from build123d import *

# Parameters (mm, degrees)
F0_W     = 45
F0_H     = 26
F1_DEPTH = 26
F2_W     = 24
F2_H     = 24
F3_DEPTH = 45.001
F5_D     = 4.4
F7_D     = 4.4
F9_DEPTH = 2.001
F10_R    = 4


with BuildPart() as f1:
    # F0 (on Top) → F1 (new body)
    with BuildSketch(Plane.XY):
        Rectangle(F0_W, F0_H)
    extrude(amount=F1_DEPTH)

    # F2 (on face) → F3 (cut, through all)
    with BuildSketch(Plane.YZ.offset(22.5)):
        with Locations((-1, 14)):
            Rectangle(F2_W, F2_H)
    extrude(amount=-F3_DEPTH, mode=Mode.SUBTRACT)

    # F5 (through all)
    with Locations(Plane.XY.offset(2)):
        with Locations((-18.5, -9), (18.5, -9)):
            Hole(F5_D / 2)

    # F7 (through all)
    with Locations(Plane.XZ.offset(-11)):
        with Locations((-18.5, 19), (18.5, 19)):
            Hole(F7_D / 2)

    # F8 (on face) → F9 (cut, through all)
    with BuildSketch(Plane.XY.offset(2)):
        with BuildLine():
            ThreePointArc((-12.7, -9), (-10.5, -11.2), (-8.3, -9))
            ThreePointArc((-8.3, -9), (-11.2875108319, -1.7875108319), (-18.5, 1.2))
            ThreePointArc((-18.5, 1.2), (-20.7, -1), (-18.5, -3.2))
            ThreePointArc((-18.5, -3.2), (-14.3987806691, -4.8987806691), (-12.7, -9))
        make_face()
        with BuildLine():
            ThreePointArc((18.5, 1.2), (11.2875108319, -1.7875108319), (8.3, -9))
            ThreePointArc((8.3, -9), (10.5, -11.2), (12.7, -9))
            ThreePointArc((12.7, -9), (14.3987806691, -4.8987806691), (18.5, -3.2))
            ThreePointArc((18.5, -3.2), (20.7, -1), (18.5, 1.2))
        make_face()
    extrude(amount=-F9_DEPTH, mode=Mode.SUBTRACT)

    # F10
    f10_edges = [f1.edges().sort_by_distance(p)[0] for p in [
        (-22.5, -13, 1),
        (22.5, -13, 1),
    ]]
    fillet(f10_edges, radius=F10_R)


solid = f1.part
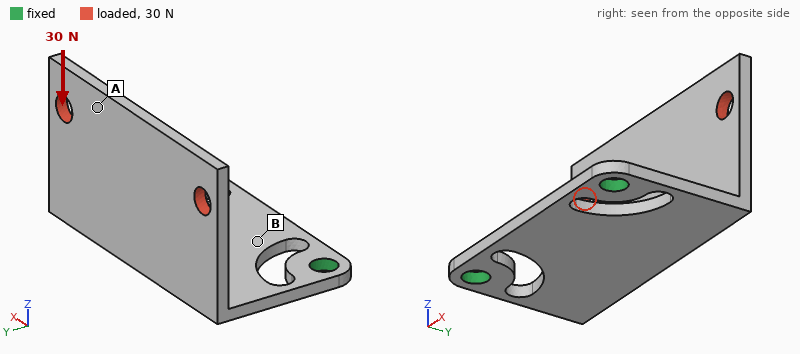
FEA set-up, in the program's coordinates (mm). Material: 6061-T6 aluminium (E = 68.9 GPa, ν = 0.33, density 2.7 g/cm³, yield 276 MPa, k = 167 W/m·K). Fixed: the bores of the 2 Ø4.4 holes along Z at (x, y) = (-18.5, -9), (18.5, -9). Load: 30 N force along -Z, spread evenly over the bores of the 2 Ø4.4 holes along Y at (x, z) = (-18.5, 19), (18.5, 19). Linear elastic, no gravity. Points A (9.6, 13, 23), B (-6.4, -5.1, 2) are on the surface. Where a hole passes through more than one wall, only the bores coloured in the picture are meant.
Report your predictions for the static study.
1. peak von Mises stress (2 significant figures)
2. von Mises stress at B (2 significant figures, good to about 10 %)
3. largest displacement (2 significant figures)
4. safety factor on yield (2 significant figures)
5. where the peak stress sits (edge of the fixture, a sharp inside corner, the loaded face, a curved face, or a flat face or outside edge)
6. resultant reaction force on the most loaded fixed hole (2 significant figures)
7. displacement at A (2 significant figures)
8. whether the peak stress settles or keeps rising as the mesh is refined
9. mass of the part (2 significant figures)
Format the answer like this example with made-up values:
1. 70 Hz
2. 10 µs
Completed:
1. 100 MPa
2. 17 MPa
3. 0.24 mm
4. 2.7
5. a curved face
6. 15 N
7. 0.22 mm
8. settles
9. 11 g
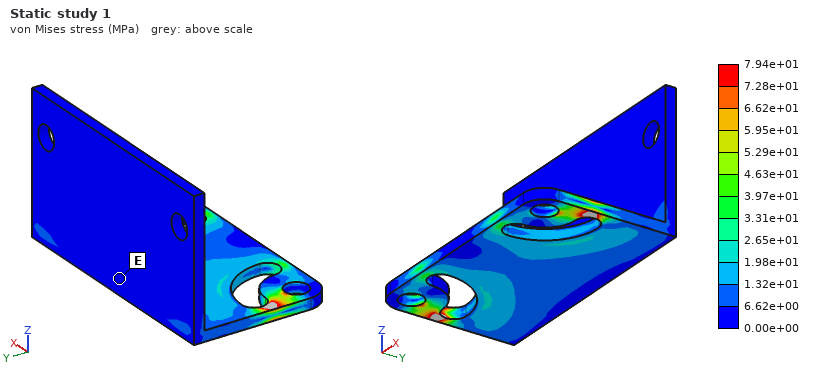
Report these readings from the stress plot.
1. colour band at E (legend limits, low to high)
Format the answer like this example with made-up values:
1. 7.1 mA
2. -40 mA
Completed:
1. 0.00e+00 to 6.62e+00 MPa
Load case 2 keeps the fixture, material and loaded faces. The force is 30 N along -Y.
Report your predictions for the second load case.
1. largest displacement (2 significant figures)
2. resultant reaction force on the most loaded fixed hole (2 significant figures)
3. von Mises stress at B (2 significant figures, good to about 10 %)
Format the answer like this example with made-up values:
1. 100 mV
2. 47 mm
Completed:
1. 0.33 mm
2. 15 N
3. 25 MPa
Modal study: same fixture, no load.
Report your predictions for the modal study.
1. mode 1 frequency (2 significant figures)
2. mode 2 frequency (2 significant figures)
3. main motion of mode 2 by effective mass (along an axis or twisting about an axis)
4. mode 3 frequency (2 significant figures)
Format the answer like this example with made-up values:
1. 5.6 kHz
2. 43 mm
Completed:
1. 700 Hz
2. 1800 Hz
3. along X
4. 2300 Hz
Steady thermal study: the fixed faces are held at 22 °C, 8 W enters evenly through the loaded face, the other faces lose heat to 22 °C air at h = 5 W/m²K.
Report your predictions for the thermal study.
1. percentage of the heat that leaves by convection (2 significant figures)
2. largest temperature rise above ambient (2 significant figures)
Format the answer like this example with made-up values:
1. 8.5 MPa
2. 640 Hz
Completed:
1. 8.0 %
2. 43 K
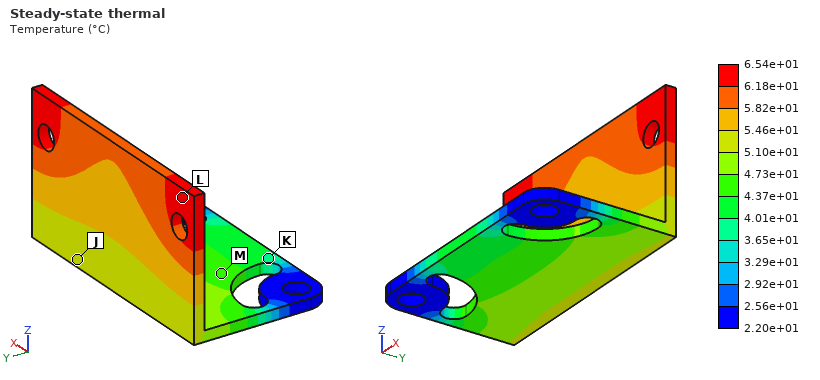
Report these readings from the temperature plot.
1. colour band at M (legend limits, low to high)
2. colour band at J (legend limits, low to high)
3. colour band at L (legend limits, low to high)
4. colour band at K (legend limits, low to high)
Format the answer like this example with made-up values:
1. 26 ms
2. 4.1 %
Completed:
1. 4.37e+01 to 4.73e+01 °C
2. 5.10e+01 to 5.46e+01 °C
3. 6.18e+01 to 6.54e+01 °C
4. 3.65e+01 to 4.01e+01 °C
